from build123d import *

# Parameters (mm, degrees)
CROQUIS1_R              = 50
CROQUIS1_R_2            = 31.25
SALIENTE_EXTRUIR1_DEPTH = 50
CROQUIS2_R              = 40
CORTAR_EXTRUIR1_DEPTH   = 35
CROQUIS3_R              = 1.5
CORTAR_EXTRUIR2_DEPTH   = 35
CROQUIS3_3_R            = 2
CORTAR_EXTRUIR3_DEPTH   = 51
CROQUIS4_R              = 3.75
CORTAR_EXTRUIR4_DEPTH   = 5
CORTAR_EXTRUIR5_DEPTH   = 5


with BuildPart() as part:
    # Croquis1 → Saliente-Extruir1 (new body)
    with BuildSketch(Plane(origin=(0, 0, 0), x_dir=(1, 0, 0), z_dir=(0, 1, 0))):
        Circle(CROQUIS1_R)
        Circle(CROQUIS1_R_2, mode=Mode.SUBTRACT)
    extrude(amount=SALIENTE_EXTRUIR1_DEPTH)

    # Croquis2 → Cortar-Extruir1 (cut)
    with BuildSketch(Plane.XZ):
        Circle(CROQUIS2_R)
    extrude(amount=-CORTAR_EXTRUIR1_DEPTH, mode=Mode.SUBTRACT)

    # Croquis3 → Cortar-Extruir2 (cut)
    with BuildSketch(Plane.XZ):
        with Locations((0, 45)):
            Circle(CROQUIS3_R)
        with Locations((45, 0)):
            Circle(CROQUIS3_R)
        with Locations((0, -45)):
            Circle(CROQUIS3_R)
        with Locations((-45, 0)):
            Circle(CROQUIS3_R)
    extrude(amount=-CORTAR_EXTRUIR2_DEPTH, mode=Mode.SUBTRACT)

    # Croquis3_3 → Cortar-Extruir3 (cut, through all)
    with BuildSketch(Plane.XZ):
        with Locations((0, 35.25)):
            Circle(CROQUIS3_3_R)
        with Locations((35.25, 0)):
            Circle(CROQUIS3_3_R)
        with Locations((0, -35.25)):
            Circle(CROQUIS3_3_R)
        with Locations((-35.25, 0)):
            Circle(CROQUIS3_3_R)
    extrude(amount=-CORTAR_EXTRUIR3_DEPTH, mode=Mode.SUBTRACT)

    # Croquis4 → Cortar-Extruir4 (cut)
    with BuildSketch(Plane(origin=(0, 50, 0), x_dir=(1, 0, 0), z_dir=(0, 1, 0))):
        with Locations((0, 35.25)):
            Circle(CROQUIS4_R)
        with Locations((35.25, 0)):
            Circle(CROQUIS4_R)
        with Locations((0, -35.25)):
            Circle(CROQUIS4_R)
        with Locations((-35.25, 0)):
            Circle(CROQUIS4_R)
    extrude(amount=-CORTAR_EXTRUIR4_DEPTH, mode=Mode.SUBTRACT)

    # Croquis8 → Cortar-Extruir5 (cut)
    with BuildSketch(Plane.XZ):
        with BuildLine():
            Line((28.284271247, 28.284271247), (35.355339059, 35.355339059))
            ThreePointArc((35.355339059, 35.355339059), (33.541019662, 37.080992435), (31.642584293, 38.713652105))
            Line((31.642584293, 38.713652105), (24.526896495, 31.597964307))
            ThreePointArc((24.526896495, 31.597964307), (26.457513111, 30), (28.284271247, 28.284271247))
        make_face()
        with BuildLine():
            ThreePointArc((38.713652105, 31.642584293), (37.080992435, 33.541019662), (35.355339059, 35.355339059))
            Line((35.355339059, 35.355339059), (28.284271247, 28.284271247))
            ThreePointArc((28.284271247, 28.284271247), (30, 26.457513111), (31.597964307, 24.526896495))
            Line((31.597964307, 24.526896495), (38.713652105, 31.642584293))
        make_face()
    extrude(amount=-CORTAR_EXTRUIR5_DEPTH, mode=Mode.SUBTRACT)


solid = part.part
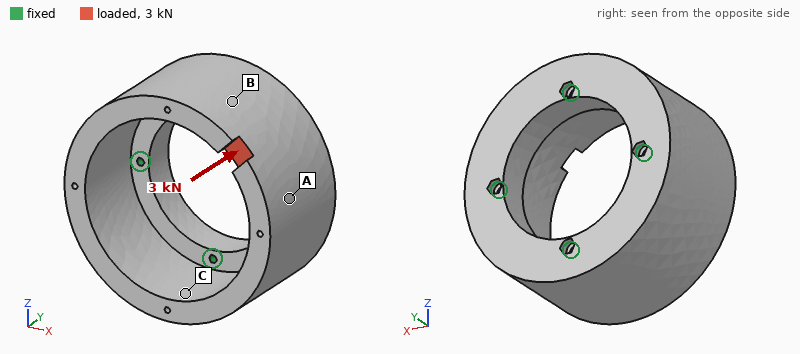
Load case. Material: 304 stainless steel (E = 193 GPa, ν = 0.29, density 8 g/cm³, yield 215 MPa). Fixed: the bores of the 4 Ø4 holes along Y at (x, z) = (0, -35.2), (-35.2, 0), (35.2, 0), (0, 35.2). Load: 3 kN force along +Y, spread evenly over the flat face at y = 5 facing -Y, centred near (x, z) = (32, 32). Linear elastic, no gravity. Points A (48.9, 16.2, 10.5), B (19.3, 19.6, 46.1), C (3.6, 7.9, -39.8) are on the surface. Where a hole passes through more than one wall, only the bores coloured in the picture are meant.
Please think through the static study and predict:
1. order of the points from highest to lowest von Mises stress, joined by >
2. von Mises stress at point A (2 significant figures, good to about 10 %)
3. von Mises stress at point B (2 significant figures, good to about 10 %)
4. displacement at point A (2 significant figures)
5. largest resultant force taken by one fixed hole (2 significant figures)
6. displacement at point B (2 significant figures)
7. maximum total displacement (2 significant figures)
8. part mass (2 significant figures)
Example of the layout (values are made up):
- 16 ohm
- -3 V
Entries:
- B > A > C
- 7.9 MPa
- 11 MPa
- 4.2 µm
- 1.9 kN
- 5.5 µm
- 10 µm
- 1.3 kg
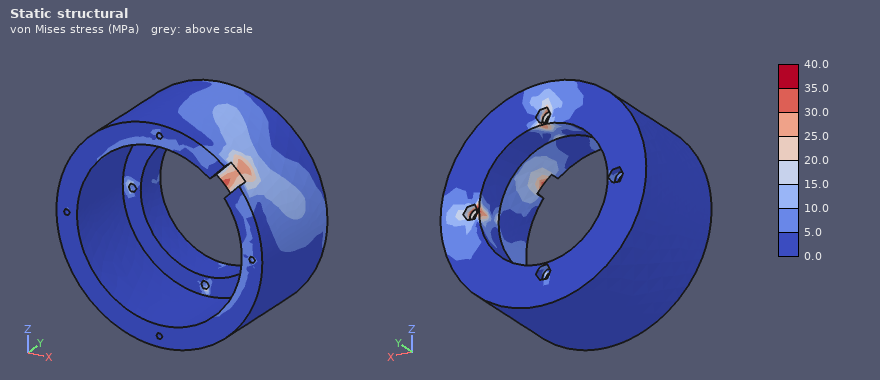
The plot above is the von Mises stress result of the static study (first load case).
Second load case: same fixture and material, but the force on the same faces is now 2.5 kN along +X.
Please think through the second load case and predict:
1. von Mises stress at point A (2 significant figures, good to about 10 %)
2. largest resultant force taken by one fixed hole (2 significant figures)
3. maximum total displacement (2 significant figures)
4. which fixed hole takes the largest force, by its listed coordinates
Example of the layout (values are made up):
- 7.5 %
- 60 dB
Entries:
- 16 MPa
- 2.0 kN
- 19 µm
- (0, 35.2)
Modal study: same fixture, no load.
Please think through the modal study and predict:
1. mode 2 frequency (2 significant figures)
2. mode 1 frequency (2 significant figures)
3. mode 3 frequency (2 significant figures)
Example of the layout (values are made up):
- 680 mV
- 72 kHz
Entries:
- 6000 Hz
- 4700 Hz
- 6000 Hz
